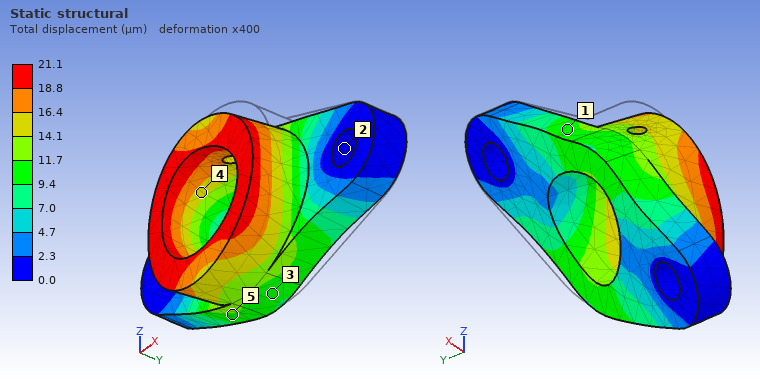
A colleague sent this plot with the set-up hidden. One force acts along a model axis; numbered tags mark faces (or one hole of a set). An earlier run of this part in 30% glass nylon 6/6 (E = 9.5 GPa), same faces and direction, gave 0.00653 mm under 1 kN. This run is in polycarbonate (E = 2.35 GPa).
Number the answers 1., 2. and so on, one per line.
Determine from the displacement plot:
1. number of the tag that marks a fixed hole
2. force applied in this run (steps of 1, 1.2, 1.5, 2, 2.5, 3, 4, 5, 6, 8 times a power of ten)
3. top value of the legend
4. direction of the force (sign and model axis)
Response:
1. 2
2. 800 N
3. 21.1 µm
4. -X
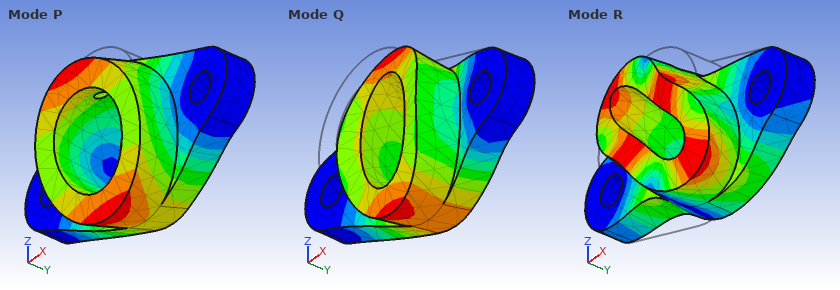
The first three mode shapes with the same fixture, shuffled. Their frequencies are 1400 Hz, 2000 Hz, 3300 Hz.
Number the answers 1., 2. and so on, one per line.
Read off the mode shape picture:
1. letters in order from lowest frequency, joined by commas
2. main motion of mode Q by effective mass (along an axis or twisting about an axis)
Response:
1. P, Q, R
2. along Y
